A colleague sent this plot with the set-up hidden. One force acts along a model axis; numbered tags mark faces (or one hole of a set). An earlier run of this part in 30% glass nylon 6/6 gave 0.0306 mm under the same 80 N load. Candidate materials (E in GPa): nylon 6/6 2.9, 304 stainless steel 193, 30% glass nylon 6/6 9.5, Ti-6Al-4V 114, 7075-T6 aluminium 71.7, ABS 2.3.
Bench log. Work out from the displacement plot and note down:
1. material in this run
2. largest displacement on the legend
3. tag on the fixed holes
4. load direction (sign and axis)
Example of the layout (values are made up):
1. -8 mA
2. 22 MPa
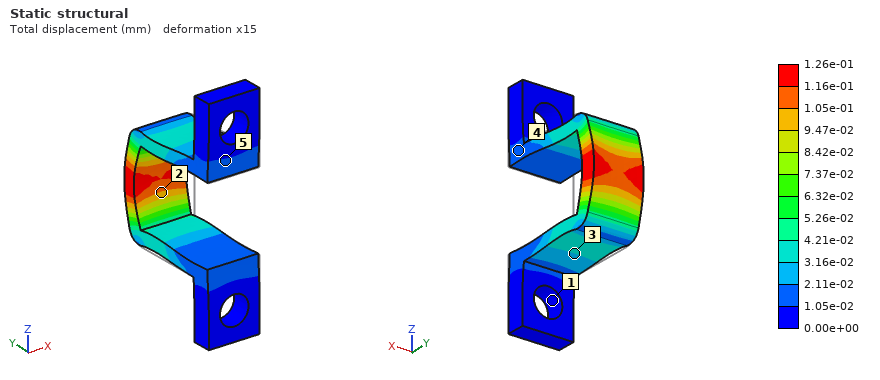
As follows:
1. ABS
2. 1.26e-01 mm
3. 1
4. +Y
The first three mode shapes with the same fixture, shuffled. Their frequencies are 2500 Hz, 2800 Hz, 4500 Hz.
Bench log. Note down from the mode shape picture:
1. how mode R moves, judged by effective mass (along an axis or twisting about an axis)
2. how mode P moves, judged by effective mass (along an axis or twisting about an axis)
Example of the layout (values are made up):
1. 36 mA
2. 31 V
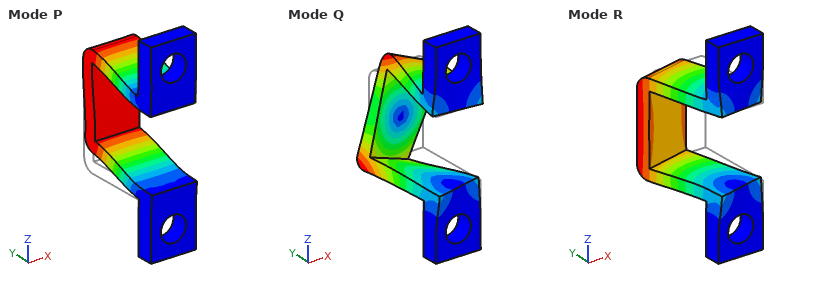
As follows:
1. along X
2. along Z
